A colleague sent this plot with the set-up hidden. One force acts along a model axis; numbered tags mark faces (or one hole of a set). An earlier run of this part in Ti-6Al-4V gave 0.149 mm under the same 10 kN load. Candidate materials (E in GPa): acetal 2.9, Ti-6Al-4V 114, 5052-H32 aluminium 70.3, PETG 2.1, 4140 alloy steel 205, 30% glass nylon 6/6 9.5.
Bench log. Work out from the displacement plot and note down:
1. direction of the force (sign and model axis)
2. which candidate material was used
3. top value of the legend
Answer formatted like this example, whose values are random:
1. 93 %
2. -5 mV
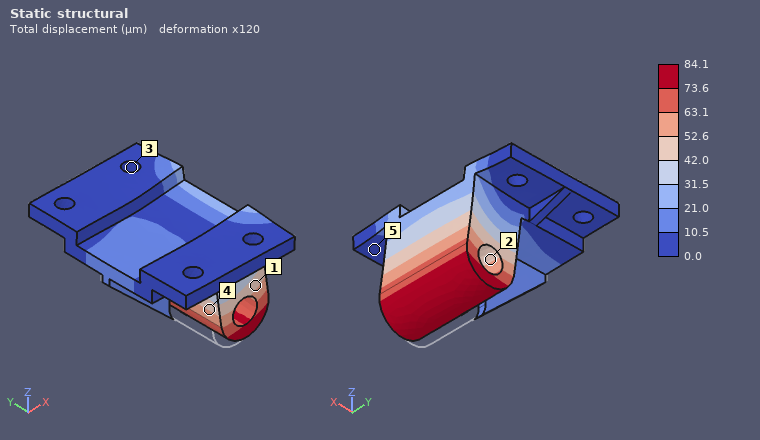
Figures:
1. +X
2. 4140 alloy steel
3. 84.1 µm
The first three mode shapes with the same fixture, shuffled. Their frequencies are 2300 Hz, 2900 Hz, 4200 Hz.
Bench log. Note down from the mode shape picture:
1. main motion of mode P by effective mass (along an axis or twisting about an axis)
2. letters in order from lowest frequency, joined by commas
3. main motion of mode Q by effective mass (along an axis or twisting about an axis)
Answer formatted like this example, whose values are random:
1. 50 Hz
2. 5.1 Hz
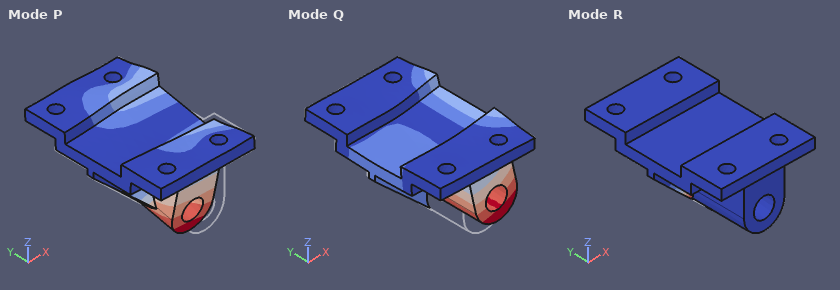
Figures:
1. along Y
2. Q, R, P
3. along X
